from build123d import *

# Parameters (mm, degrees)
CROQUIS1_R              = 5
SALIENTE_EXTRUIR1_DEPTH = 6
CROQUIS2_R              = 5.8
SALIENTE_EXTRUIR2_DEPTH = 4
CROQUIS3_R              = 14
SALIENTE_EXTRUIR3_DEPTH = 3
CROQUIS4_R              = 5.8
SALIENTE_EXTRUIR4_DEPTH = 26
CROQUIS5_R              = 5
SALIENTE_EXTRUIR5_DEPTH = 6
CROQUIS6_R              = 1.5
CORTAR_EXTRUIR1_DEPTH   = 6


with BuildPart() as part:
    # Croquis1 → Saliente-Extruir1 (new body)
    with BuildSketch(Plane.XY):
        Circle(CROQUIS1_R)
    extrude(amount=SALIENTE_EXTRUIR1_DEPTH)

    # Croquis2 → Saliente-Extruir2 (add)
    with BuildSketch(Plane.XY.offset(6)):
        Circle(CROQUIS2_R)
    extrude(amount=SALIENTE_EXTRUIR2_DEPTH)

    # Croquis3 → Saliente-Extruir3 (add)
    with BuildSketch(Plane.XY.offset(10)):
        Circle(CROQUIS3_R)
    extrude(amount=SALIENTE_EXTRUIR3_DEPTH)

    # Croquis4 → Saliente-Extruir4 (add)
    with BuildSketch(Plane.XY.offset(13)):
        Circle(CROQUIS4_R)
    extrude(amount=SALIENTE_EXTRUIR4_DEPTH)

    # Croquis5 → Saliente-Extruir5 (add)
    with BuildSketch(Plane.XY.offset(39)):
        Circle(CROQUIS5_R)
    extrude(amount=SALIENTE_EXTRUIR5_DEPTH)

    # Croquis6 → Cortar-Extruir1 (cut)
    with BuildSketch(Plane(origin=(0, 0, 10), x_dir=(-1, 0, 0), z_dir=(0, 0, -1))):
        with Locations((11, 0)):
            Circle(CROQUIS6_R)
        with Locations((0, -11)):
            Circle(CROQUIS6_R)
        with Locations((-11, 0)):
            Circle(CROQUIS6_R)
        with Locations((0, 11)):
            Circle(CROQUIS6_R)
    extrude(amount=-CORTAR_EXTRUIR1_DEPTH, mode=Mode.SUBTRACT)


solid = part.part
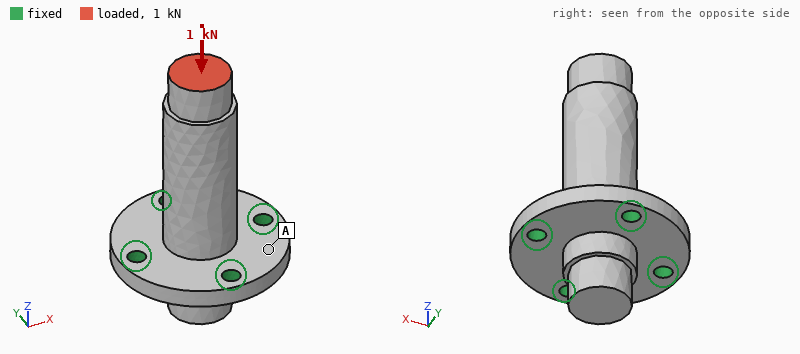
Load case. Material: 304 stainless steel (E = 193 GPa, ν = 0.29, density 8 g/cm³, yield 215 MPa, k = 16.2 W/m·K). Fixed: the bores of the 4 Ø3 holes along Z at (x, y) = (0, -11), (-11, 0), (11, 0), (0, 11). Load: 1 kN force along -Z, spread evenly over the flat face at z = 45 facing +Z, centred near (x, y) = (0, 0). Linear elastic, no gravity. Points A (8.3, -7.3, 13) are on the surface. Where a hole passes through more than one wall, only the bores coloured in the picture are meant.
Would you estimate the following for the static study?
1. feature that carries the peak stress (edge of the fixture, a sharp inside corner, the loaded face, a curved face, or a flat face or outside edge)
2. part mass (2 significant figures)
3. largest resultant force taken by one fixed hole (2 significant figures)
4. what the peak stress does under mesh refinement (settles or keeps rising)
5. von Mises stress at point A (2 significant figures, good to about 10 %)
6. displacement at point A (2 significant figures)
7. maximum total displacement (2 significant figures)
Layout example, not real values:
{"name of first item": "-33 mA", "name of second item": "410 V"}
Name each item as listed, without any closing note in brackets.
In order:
{"feature that carries the peak stress": "edge of the fixture", "part mass": "47 g", "largest resultant force taken by one fixed hole": "250 N", "what the peak stress does under mesh refinement": "keeps rising", "von Mises stress at point A": "9.1 MPa", "displacement at point A": "0.51 µm", "maximum total displacement": "3.3 µm"}
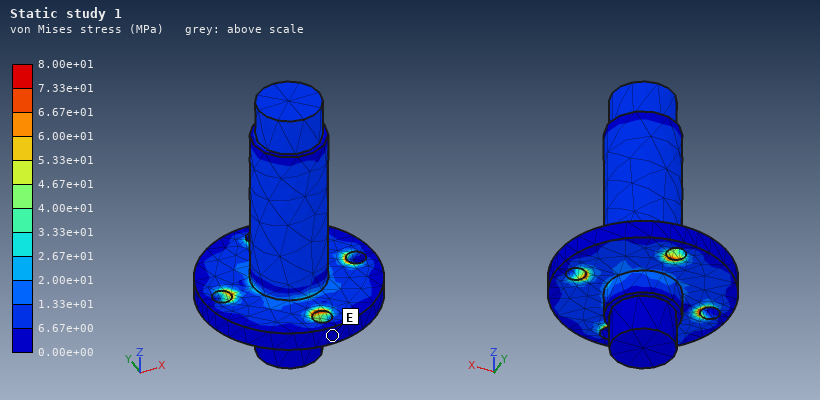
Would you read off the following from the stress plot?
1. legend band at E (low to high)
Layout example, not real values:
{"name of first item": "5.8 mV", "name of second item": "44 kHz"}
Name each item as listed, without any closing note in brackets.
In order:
{"legend band at E": "0.00e+00 to 6.67e+00 MPa"}
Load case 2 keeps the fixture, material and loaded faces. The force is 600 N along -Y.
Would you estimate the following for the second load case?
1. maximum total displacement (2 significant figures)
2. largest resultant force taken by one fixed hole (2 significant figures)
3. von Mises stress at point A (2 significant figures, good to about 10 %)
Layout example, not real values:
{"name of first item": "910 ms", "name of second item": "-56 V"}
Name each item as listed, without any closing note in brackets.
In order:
{"maximum total displacement": "74 µm", "largest resultant force taken by one fixed hole": "1.1 kN", "von Mises stress at point A": "28 MPa"}
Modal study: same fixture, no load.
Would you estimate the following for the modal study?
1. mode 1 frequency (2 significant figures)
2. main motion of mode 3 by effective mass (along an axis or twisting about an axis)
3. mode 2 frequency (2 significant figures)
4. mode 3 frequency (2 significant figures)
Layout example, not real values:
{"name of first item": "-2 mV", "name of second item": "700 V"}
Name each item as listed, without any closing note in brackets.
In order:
{"mode 1 frequency": "5400 Hz", "main motion of mode 3 by effective mass": "along Z", "mode 2 frequency": "5500 Hz", "mode 3 frequency": "19 kHz"}
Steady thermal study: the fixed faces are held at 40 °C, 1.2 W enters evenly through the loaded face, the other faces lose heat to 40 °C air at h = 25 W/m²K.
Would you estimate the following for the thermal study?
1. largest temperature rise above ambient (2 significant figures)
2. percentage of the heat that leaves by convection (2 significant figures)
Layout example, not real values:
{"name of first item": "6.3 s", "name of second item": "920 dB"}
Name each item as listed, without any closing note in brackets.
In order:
{"largest temperature rise above ambient": "23 K", "percentage of the heat that leaves by convection": "32 %"}
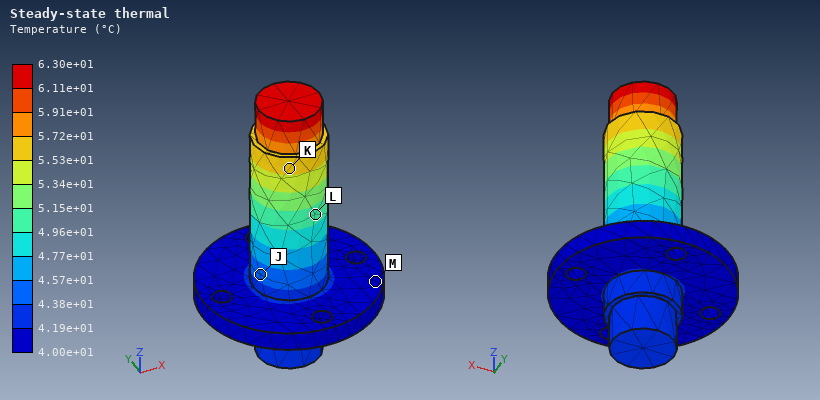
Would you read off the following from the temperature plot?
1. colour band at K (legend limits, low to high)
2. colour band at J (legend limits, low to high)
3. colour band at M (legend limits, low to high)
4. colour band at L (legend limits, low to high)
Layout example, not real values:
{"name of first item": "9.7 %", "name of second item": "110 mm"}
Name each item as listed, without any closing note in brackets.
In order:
{"colour band at K": "5.53e+01 to 5.72e+01 °C", "colour band at J": "4.38e+01 to 4.57e+01 °C", "colour band at M": "4.00e+01 to 4.19e+01 °C", "colour band at L": "4.96e+01 to 5.15e+01 °C"}
